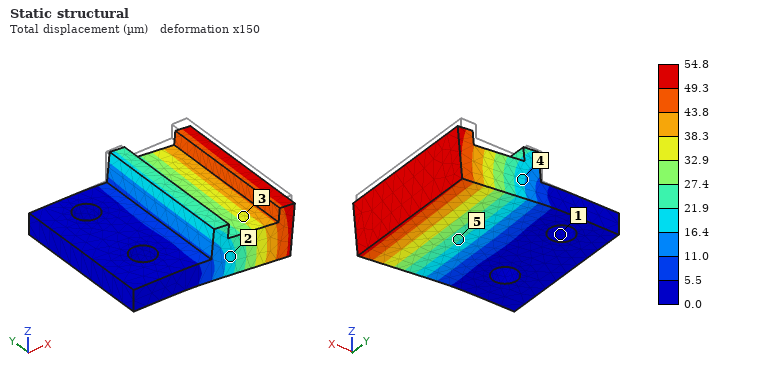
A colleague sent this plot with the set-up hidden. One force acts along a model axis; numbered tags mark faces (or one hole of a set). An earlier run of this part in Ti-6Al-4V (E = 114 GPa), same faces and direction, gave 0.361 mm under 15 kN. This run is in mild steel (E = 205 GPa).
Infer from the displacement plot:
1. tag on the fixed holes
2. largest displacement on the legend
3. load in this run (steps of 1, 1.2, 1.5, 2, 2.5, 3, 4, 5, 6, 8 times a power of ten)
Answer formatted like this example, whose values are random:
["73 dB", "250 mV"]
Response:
["1", "54.8 µm", "4 kN"]
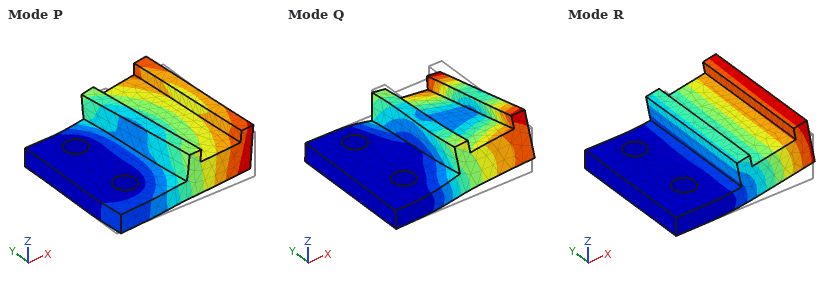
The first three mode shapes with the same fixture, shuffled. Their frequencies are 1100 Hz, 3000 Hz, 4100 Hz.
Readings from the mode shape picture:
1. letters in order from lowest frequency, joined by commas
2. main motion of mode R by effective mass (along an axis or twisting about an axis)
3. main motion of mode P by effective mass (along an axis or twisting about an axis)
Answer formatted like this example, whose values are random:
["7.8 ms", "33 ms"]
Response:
["R, Q, P", "along Z", "along Y"]
